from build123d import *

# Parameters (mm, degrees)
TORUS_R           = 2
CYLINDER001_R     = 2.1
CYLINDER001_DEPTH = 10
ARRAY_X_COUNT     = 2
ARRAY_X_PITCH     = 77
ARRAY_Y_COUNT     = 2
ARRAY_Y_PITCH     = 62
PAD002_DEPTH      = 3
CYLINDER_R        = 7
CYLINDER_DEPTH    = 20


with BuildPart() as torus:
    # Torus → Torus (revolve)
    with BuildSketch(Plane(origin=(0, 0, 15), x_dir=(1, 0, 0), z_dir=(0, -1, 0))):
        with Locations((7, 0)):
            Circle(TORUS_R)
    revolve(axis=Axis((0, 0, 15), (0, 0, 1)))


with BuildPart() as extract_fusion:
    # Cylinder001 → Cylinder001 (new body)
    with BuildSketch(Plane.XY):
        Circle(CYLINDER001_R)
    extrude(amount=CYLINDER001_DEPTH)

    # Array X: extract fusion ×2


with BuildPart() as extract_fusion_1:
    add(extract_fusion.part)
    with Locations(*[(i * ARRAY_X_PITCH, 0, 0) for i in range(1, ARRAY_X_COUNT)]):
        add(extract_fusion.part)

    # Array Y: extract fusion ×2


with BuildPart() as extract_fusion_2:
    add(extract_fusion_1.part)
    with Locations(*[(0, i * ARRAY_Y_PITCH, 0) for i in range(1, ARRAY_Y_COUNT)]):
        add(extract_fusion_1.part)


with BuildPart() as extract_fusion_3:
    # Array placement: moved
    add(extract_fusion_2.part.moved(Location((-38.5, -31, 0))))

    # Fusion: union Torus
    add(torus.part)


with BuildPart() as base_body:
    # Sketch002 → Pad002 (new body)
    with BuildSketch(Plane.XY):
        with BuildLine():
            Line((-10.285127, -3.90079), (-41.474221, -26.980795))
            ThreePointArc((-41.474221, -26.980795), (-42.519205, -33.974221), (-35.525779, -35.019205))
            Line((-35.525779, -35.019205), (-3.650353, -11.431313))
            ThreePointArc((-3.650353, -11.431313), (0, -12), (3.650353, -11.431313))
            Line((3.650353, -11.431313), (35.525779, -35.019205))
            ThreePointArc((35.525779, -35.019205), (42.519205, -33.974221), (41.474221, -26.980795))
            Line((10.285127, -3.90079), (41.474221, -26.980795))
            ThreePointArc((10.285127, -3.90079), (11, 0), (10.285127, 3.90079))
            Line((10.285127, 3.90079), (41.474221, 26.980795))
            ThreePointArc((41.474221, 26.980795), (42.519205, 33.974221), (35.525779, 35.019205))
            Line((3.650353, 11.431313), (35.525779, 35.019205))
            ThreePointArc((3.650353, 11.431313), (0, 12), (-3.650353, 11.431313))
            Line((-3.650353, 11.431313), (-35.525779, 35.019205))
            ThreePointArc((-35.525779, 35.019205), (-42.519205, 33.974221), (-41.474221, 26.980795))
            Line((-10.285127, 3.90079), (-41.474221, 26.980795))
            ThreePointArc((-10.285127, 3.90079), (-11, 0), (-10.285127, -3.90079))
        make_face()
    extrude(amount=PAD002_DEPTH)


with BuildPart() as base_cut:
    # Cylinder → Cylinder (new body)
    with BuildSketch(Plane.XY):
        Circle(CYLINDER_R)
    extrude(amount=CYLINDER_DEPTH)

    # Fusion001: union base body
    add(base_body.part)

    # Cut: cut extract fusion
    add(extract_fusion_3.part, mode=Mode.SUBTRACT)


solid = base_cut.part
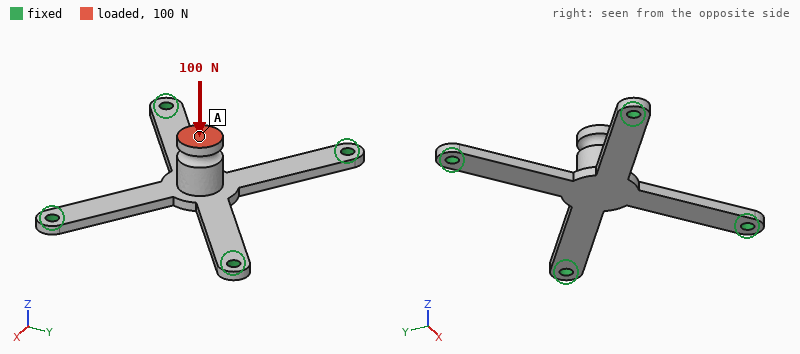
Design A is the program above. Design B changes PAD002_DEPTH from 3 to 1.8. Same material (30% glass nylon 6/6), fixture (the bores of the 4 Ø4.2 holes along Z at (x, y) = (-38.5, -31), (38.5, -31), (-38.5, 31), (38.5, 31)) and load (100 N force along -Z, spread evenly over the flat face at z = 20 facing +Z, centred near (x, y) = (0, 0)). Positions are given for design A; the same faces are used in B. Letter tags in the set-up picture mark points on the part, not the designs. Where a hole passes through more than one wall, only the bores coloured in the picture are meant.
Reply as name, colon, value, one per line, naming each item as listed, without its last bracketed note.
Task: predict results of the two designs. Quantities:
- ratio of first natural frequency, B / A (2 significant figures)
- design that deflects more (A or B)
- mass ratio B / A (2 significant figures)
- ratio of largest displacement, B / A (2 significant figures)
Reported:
ratio of first natural frequency, B / A: 0.53
design that deflects more: B
mass ratio B / A: 0.73
ratio of largest displacement, B / A: 4.3
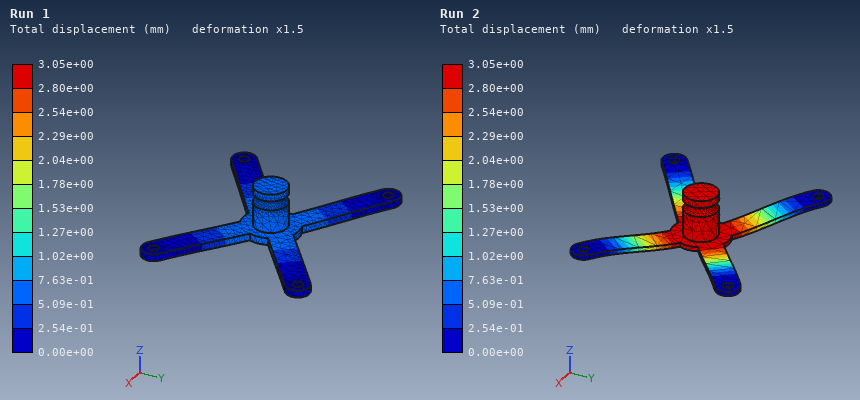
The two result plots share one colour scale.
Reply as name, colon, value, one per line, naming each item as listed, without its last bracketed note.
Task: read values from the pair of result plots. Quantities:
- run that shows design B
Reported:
run that shows design B: Run 2
